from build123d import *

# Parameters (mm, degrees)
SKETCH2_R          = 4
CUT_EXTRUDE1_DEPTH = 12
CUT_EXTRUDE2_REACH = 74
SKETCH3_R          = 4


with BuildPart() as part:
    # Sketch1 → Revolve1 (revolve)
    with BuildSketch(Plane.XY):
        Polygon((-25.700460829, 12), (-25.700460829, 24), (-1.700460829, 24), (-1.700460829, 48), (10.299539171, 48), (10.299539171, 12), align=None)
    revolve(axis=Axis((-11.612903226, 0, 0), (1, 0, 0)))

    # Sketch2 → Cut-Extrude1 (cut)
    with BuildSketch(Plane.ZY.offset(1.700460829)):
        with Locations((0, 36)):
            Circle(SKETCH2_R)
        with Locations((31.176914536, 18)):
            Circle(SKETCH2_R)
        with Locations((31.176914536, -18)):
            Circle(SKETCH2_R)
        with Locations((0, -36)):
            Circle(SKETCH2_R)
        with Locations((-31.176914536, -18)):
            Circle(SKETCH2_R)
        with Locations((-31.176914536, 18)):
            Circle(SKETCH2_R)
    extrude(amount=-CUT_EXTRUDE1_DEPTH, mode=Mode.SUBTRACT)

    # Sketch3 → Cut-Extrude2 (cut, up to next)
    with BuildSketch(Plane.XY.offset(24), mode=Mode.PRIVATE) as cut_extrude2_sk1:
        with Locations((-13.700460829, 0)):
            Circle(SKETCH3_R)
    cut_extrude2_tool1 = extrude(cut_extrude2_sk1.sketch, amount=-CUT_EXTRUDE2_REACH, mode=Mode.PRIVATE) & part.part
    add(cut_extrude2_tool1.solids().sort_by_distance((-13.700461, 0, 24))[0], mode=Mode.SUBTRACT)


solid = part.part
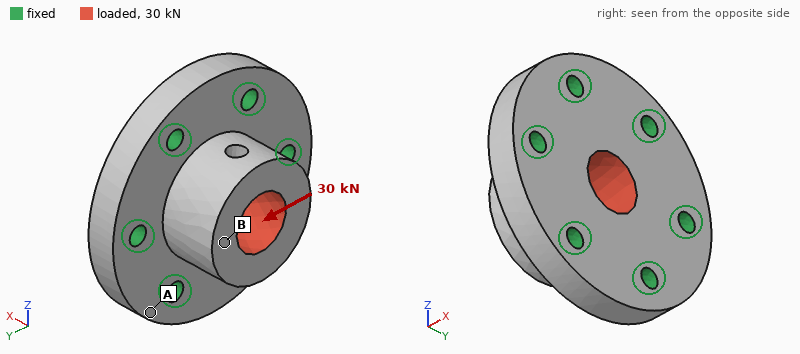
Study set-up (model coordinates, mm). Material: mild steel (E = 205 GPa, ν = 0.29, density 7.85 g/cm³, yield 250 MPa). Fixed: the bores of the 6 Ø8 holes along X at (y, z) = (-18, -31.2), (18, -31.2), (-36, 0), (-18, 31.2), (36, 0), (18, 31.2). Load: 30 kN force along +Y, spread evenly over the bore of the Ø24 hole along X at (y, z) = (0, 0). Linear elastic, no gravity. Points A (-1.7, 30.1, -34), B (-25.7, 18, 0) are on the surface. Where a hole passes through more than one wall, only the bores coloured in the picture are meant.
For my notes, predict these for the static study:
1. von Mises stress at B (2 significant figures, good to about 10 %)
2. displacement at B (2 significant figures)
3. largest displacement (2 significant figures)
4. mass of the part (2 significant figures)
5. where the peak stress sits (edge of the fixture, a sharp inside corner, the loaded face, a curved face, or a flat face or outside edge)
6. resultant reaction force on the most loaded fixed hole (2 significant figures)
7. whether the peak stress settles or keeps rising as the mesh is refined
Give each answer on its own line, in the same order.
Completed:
21 MPa
11 µm
12 µm
860 g
edge of the fixture
8.2 kN
keeps rising
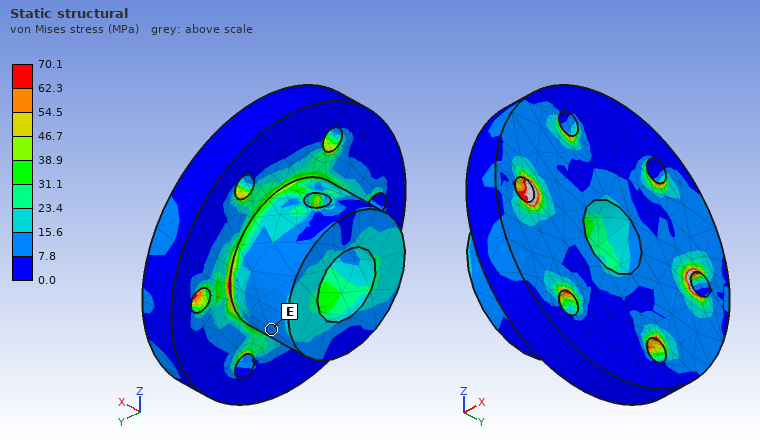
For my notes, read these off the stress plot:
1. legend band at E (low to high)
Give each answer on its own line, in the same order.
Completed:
7.8 to 15.6 MPa
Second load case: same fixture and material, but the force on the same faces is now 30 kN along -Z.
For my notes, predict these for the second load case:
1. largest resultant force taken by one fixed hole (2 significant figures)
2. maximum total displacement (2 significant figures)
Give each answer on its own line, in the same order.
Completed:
7.2 kN
11 µm
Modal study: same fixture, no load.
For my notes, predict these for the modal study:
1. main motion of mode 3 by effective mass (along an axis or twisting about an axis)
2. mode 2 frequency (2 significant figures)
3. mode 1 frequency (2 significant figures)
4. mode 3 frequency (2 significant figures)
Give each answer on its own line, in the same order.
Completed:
along X
15 kHz
15 kHz
16 kHz
